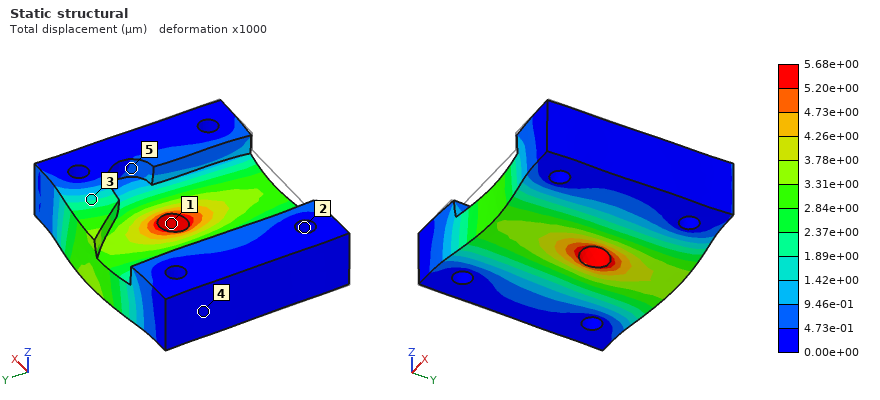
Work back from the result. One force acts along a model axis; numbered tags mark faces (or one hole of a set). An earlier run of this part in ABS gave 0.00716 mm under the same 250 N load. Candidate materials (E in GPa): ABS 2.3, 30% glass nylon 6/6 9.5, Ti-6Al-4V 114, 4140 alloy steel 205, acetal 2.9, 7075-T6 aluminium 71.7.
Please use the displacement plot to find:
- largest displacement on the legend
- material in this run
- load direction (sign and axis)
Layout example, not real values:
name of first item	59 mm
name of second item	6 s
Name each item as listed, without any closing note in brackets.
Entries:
largest displacement on the legend	5.68e+00 µm
material in this run	acetal
load direction	+Y
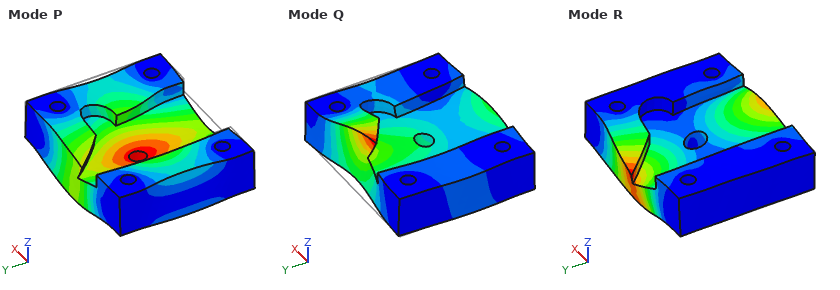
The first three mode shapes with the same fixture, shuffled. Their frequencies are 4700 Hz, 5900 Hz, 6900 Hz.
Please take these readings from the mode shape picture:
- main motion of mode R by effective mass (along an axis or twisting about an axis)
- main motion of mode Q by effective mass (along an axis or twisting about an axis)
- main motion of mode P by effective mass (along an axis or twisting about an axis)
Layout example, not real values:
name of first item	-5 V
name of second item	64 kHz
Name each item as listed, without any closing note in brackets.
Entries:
main motion of mode R by effective mass	twisting about X
main motion of mode Q by effective mass	along Y
main motion of mode P by effective mass	along Z
